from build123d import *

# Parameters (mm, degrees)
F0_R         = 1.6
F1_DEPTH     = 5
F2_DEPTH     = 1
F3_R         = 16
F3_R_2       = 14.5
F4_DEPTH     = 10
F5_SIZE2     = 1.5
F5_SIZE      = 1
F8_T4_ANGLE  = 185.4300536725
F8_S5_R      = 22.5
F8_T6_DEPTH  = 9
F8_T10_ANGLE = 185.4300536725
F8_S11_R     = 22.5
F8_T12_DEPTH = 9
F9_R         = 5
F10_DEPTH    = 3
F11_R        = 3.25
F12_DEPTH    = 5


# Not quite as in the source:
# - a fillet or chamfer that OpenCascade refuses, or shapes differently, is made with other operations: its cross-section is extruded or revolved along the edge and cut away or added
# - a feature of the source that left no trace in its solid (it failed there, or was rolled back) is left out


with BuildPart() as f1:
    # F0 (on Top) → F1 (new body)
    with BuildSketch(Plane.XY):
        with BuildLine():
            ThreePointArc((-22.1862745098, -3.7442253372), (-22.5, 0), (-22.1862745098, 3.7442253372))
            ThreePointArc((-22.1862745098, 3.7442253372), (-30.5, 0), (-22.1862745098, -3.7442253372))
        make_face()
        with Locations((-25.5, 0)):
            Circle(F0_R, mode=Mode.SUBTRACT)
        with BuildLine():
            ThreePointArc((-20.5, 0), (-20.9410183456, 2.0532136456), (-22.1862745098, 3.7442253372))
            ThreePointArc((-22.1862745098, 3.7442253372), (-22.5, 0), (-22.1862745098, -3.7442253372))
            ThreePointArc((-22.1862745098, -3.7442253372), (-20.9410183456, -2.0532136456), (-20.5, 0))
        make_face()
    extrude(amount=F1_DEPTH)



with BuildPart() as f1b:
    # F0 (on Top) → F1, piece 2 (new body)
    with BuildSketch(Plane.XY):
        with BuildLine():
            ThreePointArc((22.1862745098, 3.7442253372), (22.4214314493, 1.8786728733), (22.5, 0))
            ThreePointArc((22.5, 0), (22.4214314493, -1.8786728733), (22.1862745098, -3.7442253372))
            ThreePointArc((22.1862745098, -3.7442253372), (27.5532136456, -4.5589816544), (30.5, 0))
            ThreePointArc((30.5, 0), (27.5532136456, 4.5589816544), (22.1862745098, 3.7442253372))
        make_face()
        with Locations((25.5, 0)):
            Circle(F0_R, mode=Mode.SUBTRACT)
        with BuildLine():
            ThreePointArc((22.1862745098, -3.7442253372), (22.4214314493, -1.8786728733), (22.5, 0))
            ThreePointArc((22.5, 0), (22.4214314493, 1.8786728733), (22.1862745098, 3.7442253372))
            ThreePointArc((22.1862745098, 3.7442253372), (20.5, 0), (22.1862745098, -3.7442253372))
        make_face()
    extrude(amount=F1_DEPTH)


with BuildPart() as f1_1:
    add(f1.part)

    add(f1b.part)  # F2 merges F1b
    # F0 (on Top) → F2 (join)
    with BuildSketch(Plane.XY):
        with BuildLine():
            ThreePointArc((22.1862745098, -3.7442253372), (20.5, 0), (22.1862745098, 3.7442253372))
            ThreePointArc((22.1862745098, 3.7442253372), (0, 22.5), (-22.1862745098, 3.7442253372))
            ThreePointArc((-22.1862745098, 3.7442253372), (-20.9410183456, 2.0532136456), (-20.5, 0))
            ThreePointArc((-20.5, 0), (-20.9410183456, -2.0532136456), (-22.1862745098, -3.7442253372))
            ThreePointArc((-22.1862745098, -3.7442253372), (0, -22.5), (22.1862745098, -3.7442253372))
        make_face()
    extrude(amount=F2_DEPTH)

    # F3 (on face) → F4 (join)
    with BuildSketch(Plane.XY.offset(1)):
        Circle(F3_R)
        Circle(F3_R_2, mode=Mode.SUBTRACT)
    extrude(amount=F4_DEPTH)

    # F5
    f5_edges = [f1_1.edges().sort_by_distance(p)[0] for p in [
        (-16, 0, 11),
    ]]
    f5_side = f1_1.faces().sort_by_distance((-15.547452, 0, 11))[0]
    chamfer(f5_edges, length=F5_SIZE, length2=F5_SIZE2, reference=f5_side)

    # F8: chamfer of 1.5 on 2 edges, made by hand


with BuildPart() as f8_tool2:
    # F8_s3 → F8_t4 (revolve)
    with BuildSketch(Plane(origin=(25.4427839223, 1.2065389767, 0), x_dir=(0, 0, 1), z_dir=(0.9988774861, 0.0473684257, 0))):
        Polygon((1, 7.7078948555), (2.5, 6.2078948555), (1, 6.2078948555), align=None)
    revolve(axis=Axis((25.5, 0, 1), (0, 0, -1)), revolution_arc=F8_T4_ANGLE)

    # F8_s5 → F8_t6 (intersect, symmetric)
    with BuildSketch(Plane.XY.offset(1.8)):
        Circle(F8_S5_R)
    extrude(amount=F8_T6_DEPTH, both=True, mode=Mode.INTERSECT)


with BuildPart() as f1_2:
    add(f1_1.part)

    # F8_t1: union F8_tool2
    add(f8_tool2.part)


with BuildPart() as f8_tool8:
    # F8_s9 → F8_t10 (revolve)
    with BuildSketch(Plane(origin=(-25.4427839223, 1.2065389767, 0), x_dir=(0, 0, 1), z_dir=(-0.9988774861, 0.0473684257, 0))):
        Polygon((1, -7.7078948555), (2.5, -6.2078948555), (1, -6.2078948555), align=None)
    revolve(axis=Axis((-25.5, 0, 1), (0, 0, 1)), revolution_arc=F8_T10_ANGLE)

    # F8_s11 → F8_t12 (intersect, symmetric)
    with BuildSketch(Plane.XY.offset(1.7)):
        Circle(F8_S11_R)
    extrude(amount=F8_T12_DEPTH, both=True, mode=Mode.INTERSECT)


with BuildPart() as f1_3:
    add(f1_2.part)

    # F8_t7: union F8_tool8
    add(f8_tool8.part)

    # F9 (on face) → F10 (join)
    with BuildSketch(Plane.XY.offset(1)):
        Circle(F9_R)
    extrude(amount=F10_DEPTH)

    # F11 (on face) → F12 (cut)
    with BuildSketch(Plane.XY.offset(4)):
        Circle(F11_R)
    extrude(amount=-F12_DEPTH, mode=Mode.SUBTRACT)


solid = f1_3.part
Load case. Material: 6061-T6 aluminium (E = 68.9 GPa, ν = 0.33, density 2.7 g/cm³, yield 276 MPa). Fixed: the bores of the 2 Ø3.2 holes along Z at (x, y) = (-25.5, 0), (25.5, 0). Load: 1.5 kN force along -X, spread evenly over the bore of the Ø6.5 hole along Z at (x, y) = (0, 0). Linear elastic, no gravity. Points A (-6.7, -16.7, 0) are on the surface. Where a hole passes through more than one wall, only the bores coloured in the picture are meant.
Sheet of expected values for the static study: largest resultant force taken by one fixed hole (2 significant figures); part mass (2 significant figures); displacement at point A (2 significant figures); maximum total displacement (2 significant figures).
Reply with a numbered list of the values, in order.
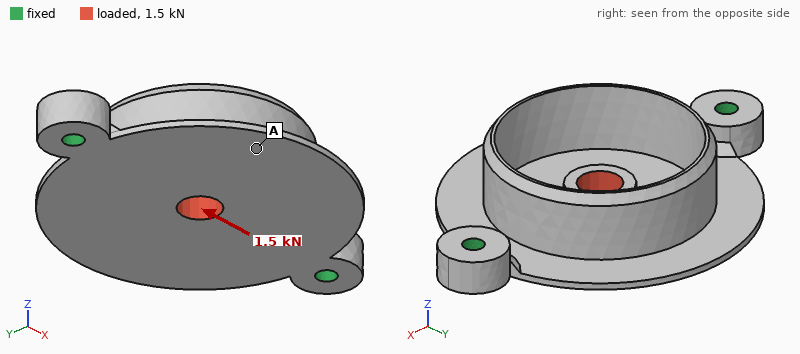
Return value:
1. 750 N
2. 10 g
3. 14 µm
4. 88 µm
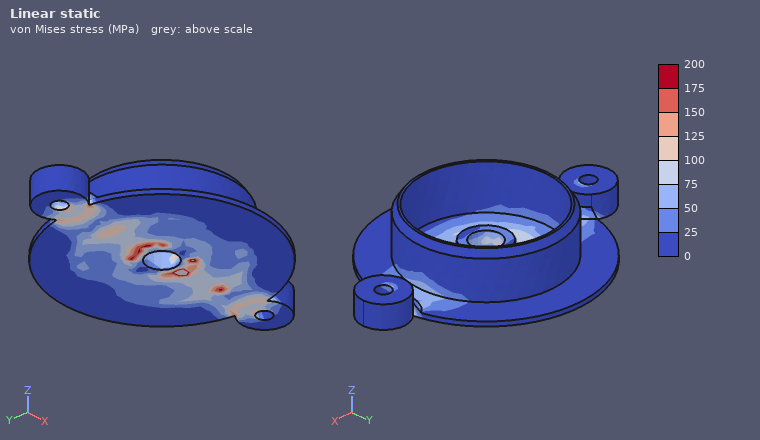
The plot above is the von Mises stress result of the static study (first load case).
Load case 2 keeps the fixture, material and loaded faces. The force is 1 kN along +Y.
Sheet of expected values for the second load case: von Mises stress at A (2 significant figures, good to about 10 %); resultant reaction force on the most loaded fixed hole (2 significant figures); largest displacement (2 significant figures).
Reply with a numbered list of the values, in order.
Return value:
1. 30 MPa
2. 500 N
3. 0.22 mm
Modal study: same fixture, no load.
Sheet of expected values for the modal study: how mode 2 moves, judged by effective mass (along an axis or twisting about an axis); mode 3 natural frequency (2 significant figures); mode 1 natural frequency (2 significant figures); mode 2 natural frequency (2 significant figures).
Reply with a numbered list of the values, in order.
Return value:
1. along Z
2. 6800 Hz
3. 1800 Hz
4. 3200 Hz
